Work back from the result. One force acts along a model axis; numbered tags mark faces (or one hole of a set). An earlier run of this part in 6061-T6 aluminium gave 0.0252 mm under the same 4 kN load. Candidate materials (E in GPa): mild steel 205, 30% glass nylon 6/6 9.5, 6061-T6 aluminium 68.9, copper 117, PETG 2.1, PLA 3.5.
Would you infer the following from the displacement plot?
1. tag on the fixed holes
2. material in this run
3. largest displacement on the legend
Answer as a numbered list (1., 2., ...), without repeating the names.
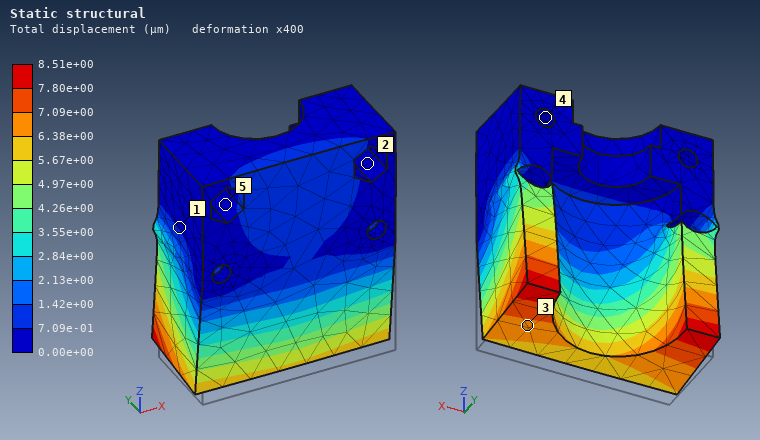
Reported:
1. 4
2. mild steel
3. 8.51e+00 µm
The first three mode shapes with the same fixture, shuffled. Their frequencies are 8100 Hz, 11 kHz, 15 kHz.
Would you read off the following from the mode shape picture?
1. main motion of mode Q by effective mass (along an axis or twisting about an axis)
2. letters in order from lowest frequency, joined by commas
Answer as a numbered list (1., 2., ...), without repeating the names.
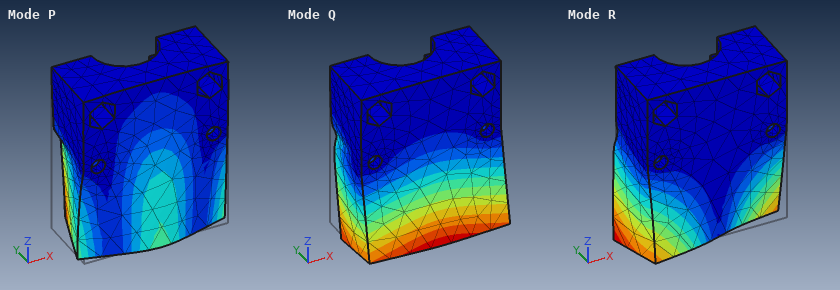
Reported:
1. along Y
2. Q, R, P
